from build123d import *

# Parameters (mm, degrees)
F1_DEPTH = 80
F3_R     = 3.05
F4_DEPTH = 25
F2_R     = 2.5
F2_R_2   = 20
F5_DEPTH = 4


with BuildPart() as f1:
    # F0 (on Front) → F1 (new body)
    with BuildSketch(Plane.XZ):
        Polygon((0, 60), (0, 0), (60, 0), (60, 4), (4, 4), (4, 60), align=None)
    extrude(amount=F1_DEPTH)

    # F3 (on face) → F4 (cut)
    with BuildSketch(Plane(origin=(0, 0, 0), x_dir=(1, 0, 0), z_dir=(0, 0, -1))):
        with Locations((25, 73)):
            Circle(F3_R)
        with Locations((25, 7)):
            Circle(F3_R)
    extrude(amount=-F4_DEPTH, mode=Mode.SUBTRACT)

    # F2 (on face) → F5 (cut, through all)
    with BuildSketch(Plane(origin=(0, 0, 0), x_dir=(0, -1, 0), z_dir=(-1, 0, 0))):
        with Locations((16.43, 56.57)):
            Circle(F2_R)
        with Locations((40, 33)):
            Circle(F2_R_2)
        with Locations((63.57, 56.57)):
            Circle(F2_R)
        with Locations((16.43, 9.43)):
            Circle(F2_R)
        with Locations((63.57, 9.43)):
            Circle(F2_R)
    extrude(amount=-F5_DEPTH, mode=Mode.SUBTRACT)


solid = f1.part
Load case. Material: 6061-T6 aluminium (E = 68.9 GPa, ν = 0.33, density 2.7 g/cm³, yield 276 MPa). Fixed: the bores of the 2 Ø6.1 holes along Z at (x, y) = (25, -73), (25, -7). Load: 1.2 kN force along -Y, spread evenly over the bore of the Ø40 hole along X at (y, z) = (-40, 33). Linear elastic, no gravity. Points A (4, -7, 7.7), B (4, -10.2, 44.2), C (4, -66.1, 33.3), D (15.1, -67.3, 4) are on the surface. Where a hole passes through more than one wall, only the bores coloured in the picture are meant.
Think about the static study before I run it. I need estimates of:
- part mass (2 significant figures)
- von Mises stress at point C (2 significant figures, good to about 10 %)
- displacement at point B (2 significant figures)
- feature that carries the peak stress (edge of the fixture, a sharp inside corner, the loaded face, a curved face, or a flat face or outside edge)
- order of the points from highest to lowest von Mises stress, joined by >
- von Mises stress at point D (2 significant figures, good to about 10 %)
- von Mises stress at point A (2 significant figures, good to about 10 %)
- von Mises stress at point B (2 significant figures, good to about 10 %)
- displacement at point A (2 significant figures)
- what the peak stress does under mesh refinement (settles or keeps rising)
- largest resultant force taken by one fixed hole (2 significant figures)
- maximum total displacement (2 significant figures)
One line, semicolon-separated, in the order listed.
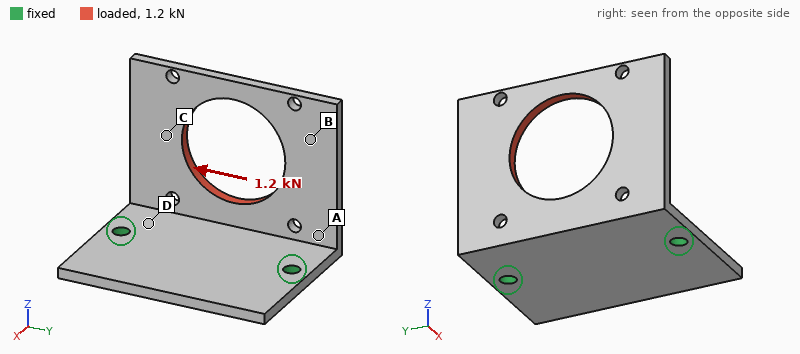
85 g; 23 MPa; 0.27 mm; edge of the fixture; D > A > C > B; 65 MPa; 49 MPa; 12 MPa; 0.13 mm; keeps rising; 920 N; 0.37 mm
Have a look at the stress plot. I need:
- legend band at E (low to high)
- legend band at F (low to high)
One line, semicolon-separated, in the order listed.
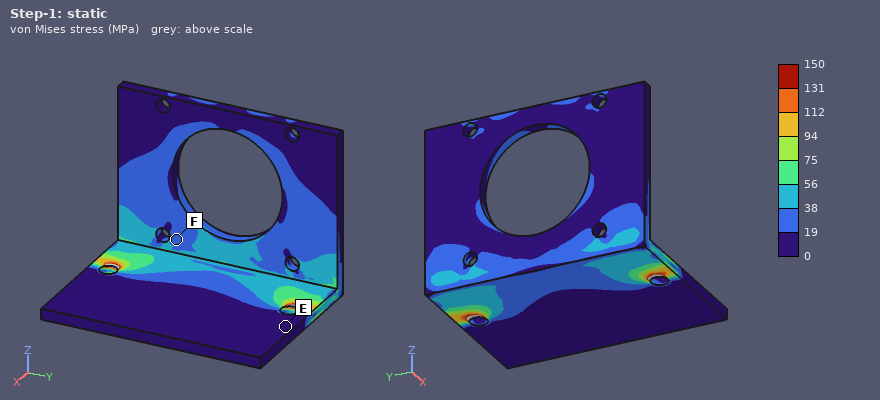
0 to 19 MPa; 19 to 38 MPa
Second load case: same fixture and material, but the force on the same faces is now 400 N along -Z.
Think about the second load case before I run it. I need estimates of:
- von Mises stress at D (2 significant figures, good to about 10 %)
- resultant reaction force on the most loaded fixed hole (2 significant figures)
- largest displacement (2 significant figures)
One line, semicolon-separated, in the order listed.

28 MPa; 200 N; 0.26 mm
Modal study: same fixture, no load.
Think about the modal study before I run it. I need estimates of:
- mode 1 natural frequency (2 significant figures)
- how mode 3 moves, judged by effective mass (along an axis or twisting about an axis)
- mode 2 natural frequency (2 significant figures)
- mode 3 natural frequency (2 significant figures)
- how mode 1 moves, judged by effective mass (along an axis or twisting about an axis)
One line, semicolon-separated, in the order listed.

620 Hz; twisting about Y; 1300 Hz; 2000 Hz; along X
